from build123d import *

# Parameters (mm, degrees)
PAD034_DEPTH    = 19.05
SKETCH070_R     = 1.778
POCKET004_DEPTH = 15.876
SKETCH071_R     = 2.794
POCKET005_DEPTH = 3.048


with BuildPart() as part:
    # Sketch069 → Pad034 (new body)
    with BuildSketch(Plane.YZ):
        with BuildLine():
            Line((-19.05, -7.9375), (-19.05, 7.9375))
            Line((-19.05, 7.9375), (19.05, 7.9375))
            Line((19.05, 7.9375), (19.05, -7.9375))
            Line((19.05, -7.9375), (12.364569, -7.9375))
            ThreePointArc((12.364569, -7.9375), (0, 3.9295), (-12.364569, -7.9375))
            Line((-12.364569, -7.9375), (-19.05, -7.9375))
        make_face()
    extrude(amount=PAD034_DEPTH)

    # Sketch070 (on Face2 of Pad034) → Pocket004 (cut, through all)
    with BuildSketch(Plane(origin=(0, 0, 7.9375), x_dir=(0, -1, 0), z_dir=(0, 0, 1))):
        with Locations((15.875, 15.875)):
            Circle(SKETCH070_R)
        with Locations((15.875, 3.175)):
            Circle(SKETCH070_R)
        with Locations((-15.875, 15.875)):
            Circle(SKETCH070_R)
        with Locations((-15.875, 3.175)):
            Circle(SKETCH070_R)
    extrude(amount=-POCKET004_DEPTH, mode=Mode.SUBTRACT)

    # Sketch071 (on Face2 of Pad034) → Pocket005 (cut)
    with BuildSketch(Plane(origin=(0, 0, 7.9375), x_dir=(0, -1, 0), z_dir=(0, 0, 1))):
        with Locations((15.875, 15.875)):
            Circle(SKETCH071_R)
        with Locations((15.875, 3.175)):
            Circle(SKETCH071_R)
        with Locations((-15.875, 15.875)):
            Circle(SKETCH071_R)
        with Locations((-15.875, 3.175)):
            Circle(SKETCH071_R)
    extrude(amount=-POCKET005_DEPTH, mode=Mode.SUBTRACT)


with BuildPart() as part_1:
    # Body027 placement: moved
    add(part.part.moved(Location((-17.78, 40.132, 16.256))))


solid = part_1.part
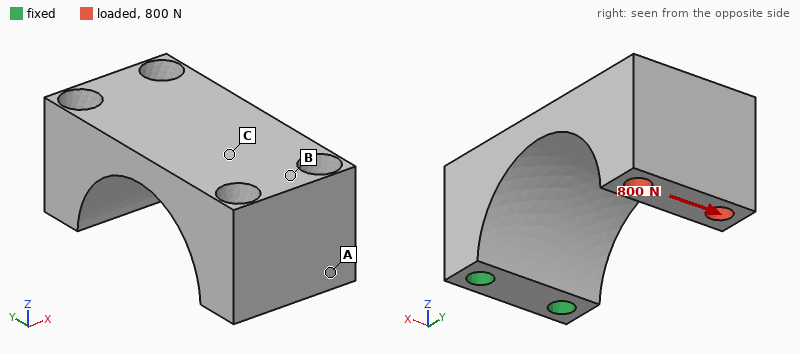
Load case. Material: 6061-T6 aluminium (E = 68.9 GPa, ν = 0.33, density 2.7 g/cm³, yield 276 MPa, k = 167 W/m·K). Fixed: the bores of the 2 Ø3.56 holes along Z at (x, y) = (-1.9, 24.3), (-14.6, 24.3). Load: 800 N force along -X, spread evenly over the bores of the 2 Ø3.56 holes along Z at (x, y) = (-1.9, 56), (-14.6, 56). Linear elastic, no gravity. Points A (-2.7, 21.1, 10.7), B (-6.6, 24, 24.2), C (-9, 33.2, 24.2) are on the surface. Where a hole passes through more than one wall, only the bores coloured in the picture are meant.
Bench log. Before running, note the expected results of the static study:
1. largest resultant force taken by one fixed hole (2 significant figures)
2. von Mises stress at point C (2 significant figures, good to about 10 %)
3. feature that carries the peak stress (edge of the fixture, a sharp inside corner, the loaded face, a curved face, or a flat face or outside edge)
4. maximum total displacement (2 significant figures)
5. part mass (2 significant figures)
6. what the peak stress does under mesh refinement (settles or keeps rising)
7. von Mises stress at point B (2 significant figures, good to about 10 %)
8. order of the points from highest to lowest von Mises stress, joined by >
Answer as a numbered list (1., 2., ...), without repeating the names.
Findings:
1. 1.8 kN
2. 45 MPa
3. edge of the fixture
4. 0.15 mm
5. 17 g
6. keeps rising
7. 28 MPa
8. C > B > A
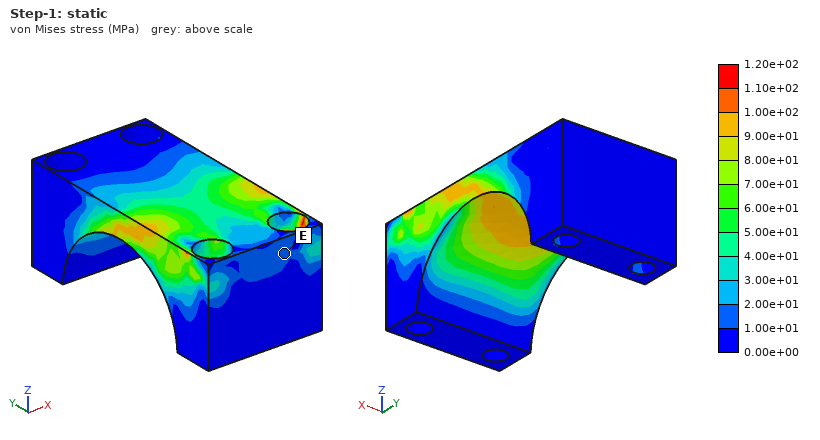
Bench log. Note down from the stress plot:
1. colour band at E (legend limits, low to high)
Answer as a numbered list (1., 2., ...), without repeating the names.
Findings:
1. 1.00e+01 to 2.00e+01 MPa
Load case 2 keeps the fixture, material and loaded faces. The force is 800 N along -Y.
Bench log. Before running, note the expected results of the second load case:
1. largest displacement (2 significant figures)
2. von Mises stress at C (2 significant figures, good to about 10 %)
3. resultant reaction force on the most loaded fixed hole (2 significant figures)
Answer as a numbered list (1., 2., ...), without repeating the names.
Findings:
1. 0.22 mm
2. 44 MPa
3. 410 N
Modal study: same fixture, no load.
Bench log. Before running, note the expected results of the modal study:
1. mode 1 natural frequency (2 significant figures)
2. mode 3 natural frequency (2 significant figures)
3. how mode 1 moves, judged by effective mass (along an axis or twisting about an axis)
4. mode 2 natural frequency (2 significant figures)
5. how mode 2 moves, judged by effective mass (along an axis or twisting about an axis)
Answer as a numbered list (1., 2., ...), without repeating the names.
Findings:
1. 2700 Hz
2. 12 kHz
3. along Z
4. 5800 Hz
5. along X
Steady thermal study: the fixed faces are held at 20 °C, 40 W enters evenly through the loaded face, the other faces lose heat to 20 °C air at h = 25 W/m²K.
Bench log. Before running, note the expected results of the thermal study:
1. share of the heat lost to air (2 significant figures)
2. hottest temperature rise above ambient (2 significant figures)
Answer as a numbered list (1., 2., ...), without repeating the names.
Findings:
1. 6.6 %
2. 71 K
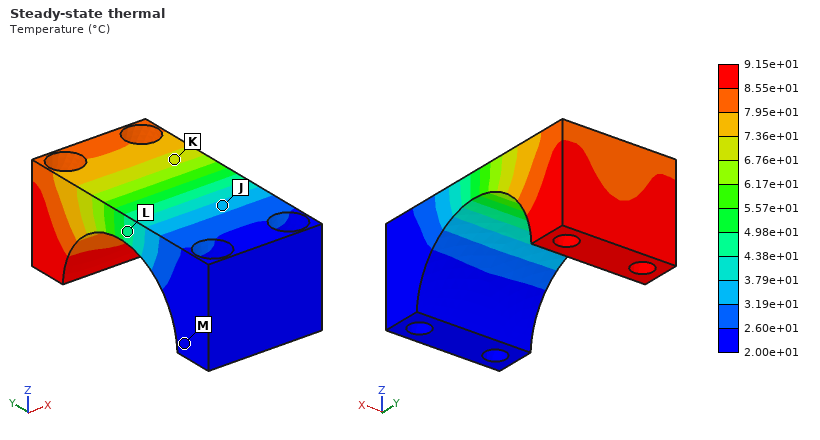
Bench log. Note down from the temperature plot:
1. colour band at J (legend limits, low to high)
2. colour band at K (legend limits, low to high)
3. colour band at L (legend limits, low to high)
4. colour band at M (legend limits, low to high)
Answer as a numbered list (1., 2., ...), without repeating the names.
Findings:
1. 3.19e+01 to 3.79e+01 °C
2. 6.76e+01 to 7.36e+01 °C
3. 4.38e+01 to 4.98e+01 °C
4. 2.00e+01 to 2.60e+01 °C
